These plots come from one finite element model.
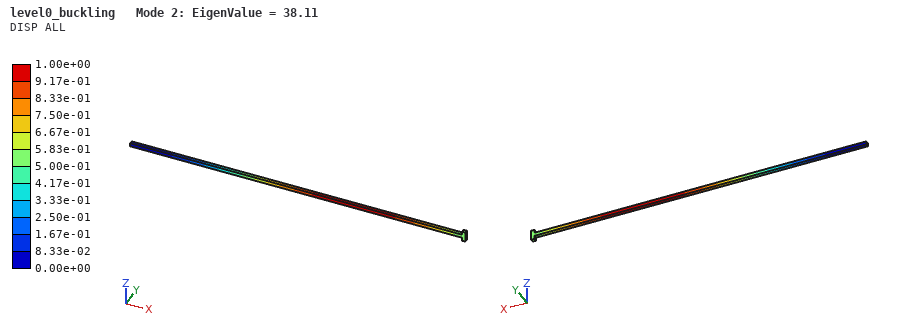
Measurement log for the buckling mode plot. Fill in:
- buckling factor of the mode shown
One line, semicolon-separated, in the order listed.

38.11
